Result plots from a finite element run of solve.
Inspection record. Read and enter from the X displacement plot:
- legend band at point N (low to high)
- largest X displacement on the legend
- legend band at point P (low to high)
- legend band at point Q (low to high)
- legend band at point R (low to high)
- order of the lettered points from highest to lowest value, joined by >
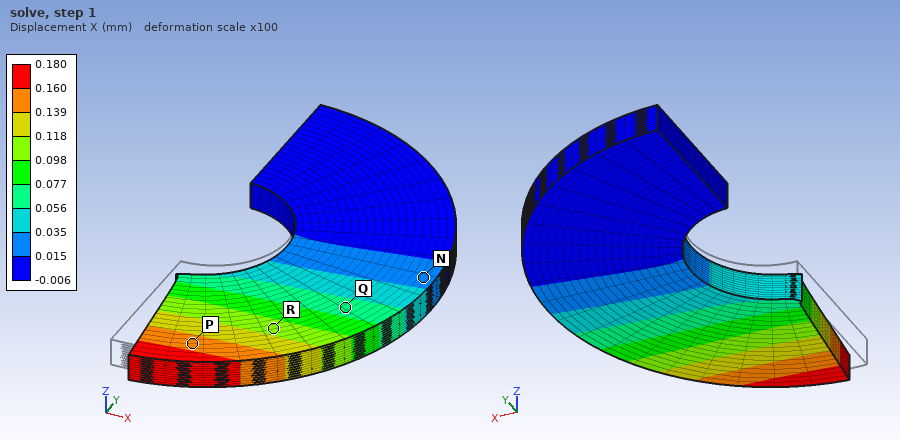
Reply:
0.015 to 0.035 mm
0.180 mm
0.139 to 0.160 mm
0.056 to 0.077 mm
0.098 to 0.118 mm
P > R > Q > N
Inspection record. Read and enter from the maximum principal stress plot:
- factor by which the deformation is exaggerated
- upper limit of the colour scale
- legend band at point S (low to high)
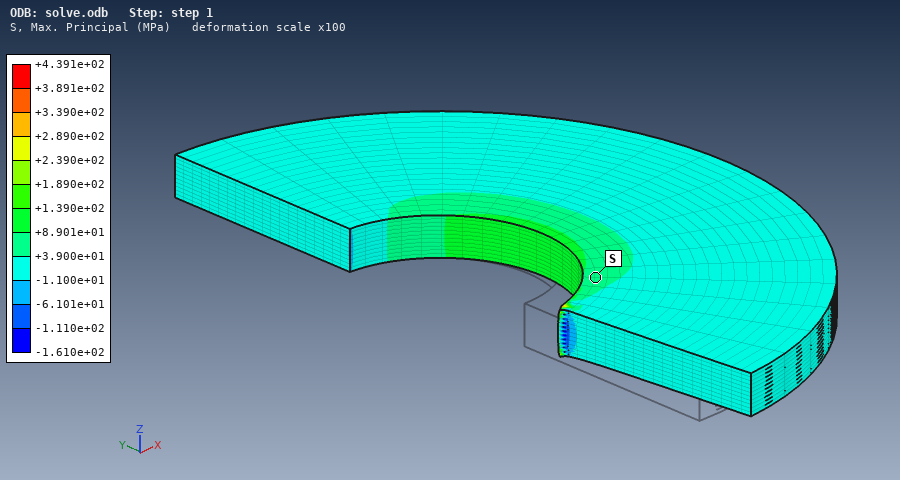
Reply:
100
+4.391e+02 MPa
+3.900e+01 to +8.901e+01 MPa
